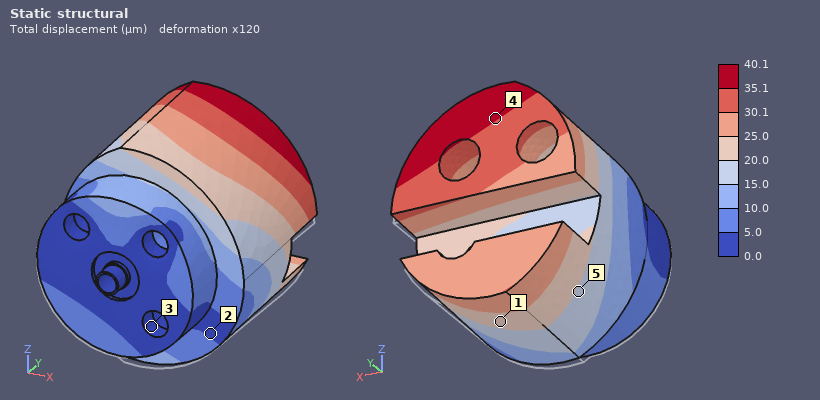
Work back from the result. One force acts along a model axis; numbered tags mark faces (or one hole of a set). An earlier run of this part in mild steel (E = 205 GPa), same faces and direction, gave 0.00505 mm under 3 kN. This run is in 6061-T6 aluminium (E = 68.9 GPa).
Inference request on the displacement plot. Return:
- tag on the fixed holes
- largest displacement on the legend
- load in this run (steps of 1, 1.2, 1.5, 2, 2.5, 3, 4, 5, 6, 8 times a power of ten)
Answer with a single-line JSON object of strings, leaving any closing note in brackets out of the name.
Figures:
{"tag on the fixed holes": "3", "largest displacement on the legend": "40.1 µm", "load in this run": "8 kN"}
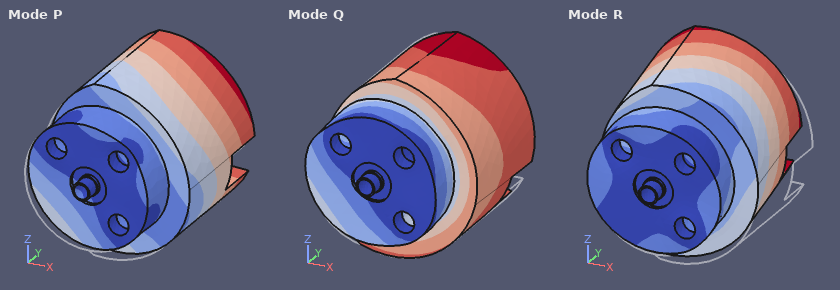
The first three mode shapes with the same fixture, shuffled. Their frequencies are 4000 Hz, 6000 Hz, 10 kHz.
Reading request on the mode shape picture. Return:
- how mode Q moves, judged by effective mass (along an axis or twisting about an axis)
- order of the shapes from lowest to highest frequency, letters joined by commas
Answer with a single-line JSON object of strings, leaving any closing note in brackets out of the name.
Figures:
{"how mode Q moves, judged by effective mass": "twisting about Y", "order of the shapes from lowest to highest frequency, letters joined by commas": "P, R, Q"}
